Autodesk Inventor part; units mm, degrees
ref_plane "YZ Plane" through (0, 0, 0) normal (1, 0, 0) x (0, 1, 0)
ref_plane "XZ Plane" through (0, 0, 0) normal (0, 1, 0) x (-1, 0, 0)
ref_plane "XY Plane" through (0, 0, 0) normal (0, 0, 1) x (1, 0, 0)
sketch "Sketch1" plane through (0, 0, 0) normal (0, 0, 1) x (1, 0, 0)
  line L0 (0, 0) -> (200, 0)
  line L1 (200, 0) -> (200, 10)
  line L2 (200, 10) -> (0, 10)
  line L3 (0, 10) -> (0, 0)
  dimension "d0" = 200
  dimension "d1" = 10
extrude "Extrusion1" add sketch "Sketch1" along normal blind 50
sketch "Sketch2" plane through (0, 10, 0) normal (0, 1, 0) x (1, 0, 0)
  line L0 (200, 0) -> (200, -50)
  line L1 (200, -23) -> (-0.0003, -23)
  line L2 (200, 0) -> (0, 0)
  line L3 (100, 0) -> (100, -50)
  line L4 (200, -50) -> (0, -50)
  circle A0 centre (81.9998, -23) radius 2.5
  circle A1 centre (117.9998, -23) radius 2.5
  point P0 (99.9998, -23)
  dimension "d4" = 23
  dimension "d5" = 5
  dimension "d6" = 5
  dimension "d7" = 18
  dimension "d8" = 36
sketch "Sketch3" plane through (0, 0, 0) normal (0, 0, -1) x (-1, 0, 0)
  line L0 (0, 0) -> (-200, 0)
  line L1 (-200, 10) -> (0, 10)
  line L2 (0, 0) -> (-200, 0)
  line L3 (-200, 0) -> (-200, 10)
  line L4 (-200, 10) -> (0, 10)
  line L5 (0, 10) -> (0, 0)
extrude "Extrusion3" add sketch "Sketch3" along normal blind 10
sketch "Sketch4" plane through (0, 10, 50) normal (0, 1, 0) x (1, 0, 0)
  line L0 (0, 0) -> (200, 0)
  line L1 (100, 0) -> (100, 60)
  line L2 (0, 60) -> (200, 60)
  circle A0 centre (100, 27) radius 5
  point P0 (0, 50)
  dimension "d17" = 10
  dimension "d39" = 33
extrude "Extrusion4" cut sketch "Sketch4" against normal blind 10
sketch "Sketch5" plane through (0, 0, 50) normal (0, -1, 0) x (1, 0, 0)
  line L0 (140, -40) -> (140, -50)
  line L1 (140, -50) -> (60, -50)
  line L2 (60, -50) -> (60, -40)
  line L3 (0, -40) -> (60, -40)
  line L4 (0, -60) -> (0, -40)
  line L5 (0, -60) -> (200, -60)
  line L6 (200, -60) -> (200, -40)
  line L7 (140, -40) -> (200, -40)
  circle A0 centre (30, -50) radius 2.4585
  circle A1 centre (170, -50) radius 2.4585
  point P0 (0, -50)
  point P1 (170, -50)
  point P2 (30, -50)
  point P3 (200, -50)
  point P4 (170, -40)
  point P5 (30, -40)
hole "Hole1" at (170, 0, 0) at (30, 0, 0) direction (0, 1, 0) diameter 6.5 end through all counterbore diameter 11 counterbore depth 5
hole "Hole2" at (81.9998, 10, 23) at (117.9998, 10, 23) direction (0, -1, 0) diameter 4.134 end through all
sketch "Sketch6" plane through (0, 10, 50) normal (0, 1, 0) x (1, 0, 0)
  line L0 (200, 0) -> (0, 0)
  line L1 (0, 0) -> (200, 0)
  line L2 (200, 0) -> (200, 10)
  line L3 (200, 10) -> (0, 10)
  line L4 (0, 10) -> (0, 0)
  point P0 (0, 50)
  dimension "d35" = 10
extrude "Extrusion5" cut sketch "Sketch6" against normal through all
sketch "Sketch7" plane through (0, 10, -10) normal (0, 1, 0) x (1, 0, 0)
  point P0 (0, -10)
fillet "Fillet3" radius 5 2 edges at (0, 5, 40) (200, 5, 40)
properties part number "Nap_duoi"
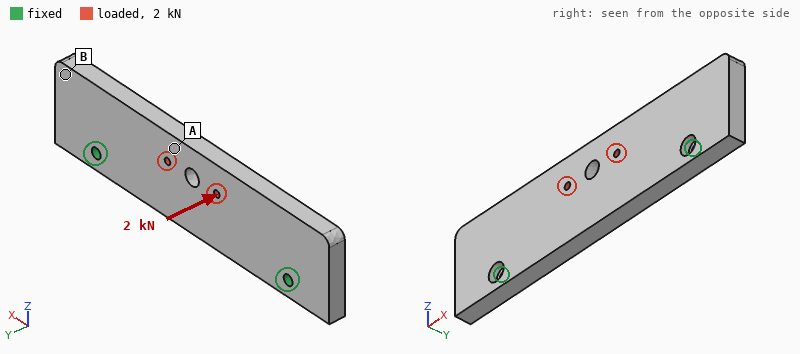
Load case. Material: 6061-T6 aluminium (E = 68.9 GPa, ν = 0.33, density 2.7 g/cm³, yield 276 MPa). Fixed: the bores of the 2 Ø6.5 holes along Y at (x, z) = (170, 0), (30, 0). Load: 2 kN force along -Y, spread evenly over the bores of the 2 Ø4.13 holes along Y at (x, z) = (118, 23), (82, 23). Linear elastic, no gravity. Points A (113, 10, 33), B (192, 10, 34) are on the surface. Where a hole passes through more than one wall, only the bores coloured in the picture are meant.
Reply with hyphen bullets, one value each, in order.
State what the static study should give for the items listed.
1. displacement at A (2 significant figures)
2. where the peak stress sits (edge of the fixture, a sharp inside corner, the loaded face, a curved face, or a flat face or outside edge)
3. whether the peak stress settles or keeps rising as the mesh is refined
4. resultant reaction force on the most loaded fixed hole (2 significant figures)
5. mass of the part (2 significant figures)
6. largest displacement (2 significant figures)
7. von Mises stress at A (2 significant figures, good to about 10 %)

- 0.28 mm
- edge of the fixture
- keeps rising
- 1.6 kN
- 260 g
- 0.32 mm
- 39 MPa
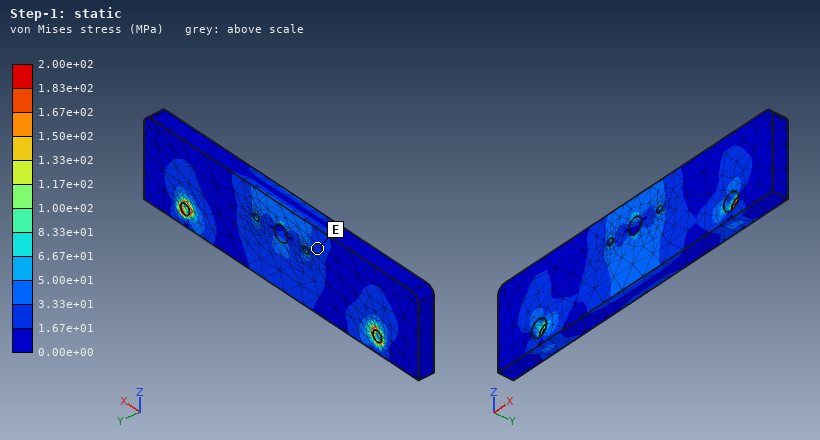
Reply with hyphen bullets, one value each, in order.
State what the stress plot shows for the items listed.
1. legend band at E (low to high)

- 1.67e+01 to 3.33e+01 MPa
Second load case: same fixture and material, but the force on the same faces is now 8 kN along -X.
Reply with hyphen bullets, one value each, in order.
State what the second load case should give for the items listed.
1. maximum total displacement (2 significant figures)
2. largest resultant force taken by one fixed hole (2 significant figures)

- 20 µm
- 4.2 kN
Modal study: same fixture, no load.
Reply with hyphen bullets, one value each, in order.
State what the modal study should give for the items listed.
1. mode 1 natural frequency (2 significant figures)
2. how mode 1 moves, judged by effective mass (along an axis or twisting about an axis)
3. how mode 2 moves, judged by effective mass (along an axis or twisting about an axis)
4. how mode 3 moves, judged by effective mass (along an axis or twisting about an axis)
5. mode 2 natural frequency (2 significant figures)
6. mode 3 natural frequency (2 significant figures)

- 1500 Hz
- along Y
- twisting about X
- twisting about Z
- 2400 Hz
- 2900 Hz
